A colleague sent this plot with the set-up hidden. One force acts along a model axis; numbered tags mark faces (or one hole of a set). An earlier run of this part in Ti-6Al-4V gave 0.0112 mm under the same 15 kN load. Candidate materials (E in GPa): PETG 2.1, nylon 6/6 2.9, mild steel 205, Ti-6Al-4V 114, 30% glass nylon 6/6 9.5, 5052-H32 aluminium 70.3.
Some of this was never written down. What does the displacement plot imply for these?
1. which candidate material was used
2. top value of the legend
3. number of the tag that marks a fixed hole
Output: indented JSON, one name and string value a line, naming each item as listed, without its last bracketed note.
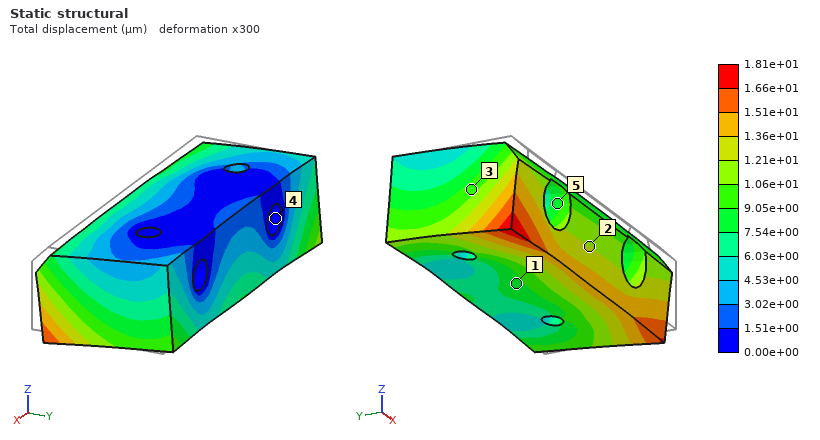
{
  "which candidate material was used": "5052-H32 aluminium",
  "top value of the legend": "1.81e+01 µm",
  "number of the tag that marks a fixed hole": "4"
}
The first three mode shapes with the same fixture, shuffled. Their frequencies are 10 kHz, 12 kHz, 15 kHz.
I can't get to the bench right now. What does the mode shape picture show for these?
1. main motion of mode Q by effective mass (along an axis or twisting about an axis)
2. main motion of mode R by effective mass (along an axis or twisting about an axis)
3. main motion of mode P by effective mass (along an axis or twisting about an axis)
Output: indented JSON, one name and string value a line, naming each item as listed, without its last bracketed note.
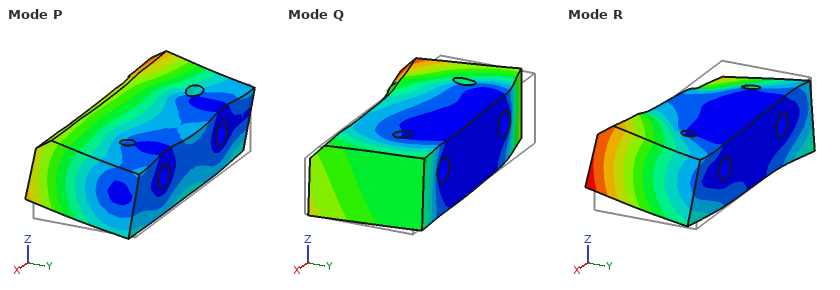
{
  "main motion of mode Q by effective mass": "along X",
  "main motion of mode R by effective mass": "twisting about Y",
  "main motion of mode P by effective mass": "along Z"
}
